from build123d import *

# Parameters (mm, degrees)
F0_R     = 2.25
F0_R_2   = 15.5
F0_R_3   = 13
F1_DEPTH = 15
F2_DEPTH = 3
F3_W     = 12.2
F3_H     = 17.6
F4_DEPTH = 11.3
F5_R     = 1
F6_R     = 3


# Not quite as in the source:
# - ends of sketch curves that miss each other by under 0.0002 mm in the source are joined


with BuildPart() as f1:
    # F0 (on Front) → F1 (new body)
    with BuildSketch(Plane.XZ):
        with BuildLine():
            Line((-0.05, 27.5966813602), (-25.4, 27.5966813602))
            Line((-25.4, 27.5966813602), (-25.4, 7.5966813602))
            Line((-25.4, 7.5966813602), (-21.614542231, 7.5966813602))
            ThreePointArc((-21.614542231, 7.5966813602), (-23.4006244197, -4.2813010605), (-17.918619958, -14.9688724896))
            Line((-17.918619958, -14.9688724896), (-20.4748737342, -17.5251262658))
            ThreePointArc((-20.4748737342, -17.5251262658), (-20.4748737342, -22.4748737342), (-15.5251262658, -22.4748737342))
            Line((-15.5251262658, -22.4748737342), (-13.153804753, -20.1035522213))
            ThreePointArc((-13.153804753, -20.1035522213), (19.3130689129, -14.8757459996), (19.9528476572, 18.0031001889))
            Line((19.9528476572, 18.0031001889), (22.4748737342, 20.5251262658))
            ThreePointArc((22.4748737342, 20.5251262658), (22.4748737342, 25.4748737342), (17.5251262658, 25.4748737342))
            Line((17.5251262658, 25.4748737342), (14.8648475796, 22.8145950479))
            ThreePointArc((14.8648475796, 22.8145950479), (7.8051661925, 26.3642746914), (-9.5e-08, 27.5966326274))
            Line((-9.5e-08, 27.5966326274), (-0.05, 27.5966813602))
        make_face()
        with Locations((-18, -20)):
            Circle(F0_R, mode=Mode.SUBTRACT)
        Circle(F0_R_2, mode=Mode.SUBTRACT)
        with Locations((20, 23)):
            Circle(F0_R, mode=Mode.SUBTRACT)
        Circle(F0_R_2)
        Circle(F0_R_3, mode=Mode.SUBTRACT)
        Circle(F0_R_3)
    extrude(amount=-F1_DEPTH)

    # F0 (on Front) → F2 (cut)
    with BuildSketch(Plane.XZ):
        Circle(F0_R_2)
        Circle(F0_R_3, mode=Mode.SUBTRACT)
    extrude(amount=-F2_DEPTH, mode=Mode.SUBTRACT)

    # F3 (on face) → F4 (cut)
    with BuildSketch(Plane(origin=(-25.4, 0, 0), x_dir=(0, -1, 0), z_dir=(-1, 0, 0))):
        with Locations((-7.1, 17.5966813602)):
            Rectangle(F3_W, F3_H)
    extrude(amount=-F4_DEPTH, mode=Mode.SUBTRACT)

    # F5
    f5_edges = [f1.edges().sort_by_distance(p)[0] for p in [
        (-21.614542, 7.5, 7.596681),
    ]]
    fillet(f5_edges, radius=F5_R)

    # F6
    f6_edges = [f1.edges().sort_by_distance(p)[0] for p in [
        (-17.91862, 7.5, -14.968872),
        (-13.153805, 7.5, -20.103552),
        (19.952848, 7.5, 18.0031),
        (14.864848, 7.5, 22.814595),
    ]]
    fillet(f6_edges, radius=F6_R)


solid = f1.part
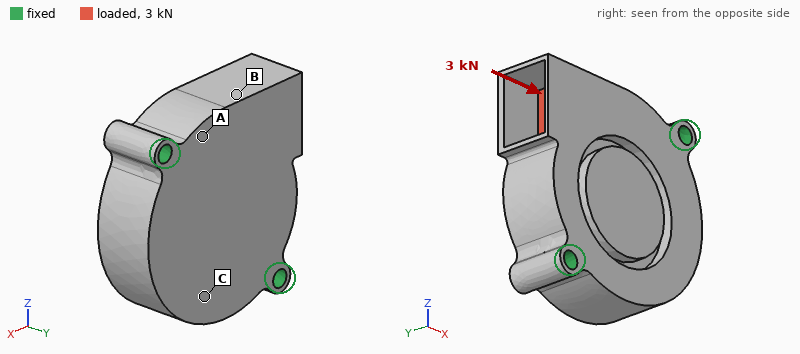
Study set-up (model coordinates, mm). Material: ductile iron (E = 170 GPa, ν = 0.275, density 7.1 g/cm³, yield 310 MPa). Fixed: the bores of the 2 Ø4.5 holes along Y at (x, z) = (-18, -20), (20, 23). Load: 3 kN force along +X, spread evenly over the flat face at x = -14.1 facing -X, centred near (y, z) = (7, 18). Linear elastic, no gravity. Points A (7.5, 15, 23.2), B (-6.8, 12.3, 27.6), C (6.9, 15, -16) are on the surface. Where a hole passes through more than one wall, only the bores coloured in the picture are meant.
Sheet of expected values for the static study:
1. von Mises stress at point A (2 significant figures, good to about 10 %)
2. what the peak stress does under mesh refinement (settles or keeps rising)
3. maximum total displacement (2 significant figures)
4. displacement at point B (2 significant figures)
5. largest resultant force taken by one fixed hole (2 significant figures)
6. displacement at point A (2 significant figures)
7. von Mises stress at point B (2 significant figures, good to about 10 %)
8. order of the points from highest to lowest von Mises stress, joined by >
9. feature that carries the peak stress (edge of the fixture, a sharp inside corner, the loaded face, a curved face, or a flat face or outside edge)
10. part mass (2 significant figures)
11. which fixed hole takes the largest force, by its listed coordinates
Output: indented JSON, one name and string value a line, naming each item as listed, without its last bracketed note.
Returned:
{
  "von Mises stress at point A": "14 MPa",
  "what the peak stress does under mesh refinement": "keeps rising",
  "maximum total displacement": "3.4 µm",
  "displacement at point B": "2.5 µm",
  "largest resultant force taken by one fixed hole": "2.4 kN",
  "displacement at point A": "1.5 µm",
  "von Mises stress at point B": "8.1 MPa",
  "order of the points from highest to lowest von Mises stress, joined by >": "A > B > C",
  "feature that carries the peak stress": "edge of the fixture",
  "part mass": "210 g",
  "which fixed hole takes the largest force, by its listed coordinates": "(20, 23)"
}
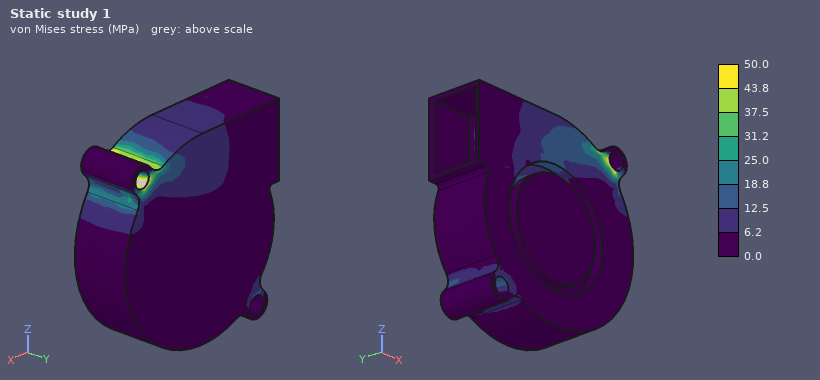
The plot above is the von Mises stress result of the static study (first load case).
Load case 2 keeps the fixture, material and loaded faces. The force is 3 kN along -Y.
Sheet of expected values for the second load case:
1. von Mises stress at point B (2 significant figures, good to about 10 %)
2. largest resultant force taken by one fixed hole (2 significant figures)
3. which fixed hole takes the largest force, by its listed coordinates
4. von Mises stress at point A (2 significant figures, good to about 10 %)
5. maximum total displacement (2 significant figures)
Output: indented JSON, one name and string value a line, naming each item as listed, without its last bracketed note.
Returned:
{
  "von Mises stress at point B": "23 MPa",
  "largest resultant force taken by one fixed hole": "1.7 kN",
  "which fixed hole takes the largest force, by its listed coordinates": "(20, 23)",
  "von Mises stress at point A": "46 MPa",
  "maximum total displacement": "57 µm"
}
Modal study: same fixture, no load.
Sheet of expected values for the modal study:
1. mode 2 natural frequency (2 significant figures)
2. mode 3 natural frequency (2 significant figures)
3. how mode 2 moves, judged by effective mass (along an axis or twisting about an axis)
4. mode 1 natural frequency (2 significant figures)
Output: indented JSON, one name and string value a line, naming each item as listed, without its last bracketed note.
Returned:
{
  "mode 2 natural frequency": "10 kHz",
  "mode 3 natural frequency": "15 kHz",
  "how mode 2 moves, judged by effective mass": "along Y",
  "mode 1 natural frequency": "6700 Hz"
}
